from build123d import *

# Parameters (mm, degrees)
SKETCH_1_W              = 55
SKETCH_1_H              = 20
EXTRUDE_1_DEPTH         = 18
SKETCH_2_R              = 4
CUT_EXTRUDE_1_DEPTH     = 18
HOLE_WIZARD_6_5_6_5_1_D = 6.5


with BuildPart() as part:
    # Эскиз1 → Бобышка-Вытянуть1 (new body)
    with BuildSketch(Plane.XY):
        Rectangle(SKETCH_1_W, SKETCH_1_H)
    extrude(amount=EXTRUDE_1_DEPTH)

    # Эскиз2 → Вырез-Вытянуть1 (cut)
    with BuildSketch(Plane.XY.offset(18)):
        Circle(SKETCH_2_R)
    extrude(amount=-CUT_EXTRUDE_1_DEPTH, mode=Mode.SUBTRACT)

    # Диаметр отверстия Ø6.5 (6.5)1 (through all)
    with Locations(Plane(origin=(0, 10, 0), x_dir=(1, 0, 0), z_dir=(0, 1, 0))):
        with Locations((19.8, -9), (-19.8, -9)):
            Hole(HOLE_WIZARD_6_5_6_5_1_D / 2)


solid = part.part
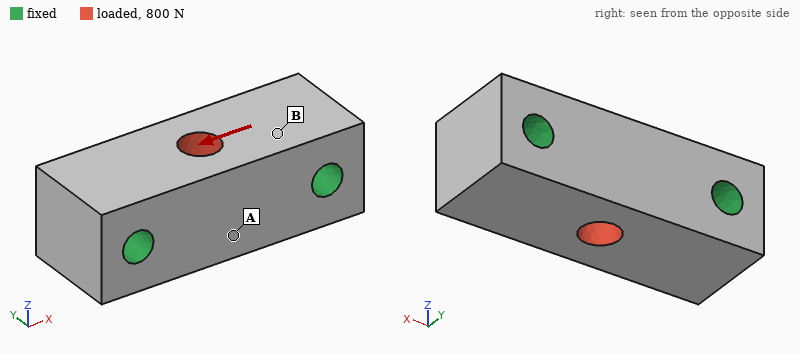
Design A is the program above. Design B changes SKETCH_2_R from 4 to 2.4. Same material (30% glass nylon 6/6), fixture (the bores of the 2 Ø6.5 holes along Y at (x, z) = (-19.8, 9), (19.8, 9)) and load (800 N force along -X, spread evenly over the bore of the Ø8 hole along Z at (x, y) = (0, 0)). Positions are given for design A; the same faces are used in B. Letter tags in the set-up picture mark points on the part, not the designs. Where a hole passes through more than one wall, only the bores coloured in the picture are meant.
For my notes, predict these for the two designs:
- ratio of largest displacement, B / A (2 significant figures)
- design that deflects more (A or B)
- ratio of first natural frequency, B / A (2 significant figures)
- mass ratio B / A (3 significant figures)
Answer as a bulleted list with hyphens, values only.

- 1.2
- B
- 0.99
- 1.03
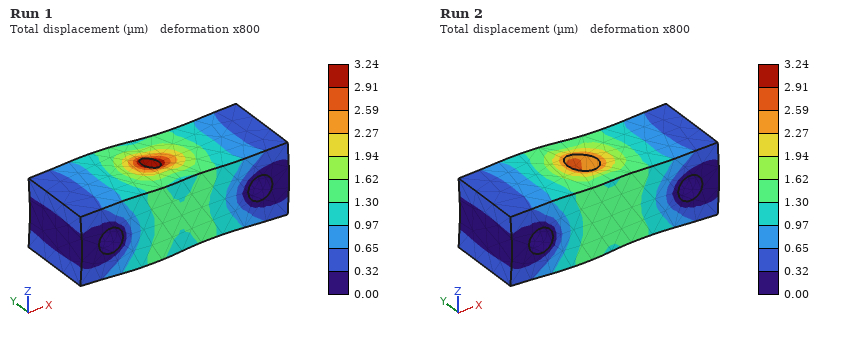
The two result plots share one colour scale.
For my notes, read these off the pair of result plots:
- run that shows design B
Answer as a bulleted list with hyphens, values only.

- Run 1
